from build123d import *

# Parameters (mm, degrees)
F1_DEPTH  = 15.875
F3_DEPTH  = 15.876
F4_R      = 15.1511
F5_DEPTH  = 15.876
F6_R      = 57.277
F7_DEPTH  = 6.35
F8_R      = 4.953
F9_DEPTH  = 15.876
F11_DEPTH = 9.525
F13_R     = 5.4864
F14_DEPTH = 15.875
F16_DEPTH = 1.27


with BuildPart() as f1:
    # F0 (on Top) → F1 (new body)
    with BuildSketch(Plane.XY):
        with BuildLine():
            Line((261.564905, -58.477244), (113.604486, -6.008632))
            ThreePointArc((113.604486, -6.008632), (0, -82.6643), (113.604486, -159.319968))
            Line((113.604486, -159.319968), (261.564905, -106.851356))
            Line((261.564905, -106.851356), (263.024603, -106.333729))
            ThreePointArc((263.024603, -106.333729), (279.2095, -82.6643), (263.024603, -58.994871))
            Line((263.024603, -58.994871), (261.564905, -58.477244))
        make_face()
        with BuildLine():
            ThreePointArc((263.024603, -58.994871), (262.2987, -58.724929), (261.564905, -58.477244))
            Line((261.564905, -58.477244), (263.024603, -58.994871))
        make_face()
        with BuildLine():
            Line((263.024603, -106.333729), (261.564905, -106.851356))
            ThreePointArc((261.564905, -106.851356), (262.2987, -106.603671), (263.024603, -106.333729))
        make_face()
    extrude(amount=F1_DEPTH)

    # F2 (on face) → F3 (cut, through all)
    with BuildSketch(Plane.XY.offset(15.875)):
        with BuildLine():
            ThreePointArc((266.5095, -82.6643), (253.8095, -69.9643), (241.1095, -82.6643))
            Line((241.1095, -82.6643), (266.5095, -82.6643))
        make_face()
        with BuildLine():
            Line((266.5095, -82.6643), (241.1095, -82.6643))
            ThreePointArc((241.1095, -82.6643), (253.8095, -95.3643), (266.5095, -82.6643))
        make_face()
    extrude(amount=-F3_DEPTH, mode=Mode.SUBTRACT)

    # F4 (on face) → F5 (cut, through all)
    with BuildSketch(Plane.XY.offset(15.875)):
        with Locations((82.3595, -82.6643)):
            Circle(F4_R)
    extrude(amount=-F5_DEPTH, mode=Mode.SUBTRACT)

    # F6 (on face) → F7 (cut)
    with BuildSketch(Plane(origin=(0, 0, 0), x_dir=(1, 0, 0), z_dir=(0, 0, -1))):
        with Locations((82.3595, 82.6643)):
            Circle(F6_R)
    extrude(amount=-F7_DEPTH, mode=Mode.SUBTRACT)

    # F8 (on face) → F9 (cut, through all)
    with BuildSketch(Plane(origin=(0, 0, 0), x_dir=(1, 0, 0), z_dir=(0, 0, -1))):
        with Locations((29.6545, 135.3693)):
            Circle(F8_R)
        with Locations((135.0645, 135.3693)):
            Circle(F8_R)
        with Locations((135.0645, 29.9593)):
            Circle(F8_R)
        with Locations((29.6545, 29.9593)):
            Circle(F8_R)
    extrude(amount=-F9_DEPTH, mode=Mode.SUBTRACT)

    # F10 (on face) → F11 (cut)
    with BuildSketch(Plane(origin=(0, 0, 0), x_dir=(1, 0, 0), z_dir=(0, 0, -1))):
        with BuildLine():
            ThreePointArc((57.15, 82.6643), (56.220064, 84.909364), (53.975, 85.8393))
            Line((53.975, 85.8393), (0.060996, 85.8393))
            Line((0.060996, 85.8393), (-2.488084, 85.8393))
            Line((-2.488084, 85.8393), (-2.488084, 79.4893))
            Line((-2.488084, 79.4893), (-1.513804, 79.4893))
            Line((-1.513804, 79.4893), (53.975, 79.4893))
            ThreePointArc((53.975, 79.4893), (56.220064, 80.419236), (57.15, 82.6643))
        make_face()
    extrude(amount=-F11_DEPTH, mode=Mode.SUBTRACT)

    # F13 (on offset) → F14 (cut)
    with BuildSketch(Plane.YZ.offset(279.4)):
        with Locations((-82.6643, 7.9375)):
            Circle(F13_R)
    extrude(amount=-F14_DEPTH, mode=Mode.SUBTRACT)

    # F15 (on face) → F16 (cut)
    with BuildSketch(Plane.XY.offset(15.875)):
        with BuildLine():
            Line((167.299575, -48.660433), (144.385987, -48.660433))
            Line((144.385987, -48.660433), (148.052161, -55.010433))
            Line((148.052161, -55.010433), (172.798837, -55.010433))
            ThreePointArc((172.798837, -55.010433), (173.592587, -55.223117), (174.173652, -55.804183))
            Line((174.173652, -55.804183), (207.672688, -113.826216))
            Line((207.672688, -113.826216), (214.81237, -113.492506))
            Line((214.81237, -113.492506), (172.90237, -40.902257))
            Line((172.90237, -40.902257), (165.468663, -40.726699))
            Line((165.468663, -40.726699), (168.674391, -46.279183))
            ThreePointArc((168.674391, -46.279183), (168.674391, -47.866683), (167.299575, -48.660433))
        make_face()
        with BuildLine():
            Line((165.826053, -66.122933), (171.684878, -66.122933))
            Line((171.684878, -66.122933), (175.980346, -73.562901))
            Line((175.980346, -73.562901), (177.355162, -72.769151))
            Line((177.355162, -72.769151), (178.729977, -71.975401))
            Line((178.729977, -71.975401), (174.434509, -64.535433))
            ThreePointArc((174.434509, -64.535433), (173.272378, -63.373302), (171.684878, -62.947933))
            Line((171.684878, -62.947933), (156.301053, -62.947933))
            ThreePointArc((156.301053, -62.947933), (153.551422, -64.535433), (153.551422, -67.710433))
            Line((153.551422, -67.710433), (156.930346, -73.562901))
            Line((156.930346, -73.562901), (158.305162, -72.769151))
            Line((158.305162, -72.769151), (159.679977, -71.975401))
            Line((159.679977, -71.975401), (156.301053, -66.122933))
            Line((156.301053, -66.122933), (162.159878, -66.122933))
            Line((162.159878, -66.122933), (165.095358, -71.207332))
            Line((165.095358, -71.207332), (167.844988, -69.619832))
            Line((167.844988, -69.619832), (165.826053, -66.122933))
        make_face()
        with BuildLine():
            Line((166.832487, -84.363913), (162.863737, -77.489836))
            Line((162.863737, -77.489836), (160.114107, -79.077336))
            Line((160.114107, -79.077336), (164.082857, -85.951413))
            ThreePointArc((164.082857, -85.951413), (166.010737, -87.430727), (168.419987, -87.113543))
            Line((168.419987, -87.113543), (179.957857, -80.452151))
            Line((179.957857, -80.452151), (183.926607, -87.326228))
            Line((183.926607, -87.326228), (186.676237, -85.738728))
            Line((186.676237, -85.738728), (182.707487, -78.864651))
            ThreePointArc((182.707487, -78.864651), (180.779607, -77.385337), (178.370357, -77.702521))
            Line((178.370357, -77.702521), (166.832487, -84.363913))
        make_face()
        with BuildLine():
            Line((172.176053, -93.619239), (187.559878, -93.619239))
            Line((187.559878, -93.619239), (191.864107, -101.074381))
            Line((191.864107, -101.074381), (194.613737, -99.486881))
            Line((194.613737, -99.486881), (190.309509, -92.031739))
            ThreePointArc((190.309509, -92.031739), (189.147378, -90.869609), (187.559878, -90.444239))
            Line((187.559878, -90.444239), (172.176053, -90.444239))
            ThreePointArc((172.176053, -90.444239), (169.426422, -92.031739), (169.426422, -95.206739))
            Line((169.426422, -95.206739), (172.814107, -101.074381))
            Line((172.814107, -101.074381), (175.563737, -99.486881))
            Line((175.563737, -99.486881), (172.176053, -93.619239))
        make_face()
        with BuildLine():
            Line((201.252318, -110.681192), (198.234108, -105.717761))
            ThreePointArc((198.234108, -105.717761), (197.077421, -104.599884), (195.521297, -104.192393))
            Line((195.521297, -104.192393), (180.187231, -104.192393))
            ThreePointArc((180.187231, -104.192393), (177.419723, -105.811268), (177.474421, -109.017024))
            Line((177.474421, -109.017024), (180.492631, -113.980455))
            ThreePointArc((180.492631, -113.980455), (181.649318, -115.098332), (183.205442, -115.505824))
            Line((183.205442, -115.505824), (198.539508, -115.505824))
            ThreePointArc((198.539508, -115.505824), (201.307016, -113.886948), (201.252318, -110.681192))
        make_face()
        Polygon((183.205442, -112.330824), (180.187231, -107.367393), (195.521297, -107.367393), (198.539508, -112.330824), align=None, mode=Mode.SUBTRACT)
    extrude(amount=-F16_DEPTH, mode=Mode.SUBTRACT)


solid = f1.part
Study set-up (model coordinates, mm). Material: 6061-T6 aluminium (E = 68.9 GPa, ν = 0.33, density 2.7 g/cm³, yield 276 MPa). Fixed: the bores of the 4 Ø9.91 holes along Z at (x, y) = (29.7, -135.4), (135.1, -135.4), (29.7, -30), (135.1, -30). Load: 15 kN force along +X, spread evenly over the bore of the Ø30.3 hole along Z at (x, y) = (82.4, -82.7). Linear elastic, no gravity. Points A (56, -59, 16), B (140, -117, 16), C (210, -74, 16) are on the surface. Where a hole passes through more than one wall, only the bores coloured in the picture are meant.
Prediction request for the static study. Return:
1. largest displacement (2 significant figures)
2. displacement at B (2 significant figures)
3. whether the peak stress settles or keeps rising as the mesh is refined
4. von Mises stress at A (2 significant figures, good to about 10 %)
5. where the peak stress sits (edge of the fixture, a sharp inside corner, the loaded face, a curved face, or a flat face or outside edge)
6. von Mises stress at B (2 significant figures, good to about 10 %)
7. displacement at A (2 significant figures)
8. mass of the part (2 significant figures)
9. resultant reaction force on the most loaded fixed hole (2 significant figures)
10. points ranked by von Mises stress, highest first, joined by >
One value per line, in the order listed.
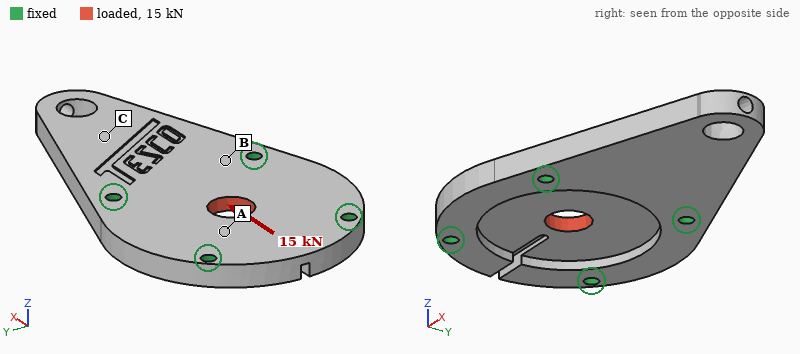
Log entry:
16 µm
3.6 µm
keeps rising
11 MPa
edge of the fixture
6.7 MPa
7.4 µm
1.1 kg
4.2 kN
A > B > C
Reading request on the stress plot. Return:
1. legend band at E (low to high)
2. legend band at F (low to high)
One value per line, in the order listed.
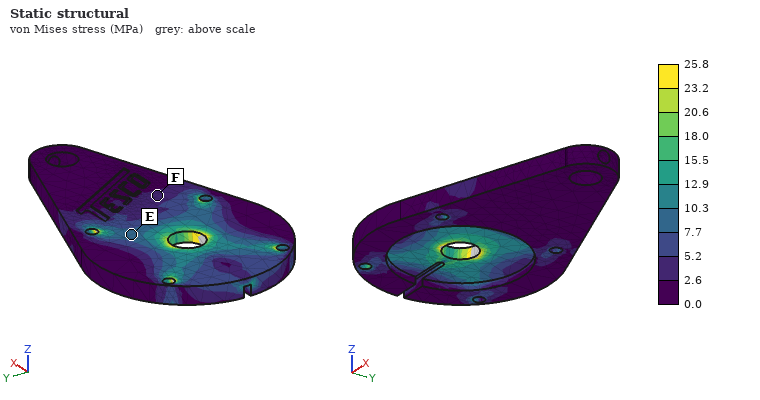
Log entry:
7.7 to 10.3 MPa
2.6 to 5.2 MPa
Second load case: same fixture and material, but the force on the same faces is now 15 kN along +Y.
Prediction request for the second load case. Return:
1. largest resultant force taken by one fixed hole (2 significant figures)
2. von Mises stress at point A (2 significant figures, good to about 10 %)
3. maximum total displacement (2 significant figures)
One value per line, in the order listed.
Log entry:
4.0 kN
10 MPa
14 µm
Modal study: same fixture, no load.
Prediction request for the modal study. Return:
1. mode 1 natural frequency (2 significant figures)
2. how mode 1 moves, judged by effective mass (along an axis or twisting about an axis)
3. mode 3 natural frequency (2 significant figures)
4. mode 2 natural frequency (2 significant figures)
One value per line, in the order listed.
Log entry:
850 Hz
along Z
3800 Hz
3400 Hz
